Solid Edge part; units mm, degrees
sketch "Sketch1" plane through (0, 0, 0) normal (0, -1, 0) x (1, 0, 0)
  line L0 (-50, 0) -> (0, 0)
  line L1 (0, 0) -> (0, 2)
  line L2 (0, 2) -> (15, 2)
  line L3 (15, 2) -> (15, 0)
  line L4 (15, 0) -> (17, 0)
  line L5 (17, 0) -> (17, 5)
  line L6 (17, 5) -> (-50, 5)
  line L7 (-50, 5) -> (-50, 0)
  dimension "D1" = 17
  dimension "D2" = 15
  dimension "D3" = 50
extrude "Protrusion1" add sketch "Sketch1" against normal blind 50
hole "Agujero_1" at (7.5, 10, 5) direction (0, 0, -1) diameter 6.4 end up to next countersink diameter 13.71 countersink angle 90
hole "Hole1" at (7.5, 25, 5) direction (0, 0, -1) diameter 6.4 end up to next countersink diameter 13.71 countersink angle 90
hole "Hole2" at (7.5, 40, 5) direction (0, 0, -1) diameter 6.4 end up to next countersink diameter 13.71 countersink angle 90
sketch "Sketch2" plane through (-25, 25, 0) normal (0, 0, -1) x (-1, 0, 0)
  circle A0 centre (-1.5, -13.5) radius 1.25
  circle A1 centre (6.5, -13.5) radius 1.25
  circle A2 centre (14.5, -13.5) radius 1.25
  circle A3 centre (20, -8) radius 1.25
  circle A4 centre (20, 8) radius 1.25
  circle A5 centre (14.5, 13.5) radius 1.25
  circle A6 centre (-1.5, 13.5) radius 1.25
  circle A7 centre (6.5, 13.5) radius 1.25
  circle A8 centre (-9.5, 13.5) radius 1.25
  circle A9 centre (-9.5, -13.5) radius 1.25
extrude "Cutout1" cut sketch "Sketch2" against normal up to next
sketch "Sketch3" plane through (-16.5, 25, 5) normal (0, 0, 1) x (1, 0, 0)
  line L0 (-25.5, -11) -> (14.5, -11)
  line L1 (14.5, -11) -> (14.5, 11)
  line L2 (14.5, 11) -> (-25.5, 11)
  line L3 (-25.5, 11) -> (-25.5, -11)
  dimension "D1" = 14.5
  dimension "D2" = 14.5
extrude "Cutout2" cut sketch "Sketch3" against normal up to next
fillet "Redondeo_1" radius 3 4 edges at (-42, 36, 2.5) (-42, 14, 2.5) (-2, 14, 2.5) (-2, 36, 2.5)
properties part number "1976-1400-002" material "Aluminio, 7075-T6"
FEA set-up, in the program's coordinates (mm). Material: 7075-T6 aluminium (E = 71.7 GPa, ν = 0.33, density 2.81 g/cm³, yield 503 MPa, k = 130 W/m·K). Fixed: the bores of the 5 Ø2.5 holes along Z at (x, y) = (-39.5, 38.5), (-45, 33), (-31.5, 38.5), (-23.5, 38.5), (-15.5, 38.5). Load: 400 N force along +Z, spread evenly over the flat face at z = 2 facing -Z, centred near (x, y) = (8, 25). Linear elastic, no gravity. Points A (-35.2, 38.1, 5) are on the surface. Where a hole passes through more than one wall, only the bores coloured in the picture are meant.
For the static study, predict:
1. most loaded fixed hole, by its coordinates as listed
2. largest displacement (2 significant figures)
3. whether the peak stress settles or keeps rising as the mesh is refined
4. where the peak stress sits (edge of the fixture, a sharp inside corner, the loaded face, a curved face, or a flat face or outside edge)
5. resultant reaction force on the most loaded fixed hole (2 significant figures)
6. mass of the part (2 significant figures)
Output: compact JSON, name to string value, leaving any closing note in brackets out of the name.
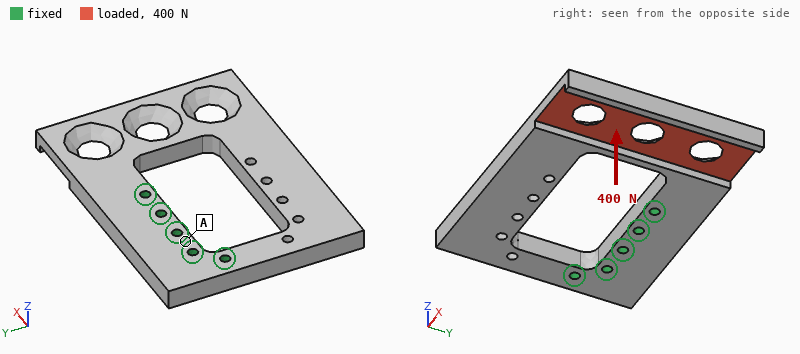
{"most loaded fixed hole, by its coordinates as listed": "(-15.5, 38.5)", "largest displacement": "0.89 mm", "whether the peak stress settles or keeps rising as the mesh is refined": "keeps rising", "where the peak stress sits": "edge of the fixture", "resultant reaction force on the most loaded fixed hole": "680 N", "mass of the part": "28 g"}
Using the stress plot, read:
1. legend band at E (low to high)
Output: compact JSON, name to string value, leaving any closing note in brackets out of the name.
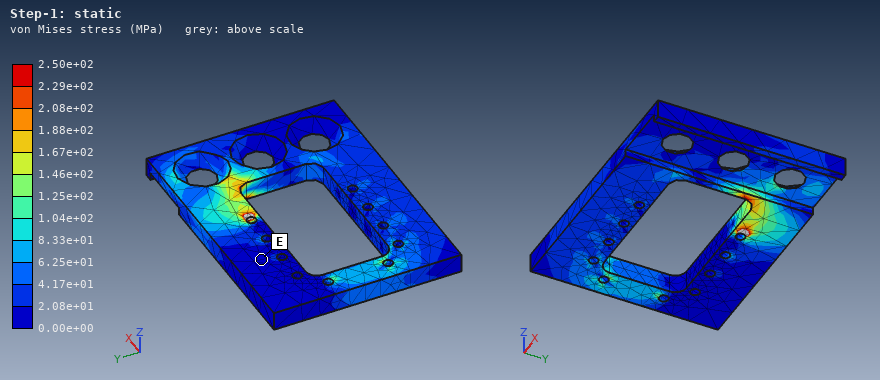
{"legend band at E": "0.00e+00 to 2.08e+01 MPa"}
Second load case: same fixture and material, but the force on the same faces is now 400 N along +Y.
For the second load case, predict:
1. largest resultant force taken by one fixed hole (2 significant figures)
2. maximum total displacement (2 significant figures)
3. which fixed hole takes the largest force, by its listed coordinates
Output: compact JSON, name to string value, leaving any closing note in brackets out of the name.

{"largest resultant force taken by one fixed hole": "820 N", "maximum total displacement": "55 µm", "which fixed hole takes the largest force, by its listed coordinates": "(-15.5, 38.5)"}
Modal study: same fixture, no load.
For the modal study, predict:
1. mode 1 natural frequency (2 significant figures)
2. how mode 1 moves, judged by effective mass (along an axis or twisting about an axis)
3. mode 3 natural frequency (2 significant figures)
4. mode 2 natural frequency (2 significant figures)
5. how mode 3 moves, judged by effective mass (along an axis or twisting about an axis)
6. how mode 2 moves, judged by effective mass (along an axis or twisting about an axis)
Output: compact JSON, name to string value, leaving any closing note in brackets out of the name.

{"mode 1 natural frequency": "1200 Hz", "how mode 1 moves, judged by effective mass": "along Z", "mode 3 natural frequency": "4000 Hz", "mode 2 natural frequency": "2600 Hz", "how mode 3 moves, judged by effective mass": "along X", "how mode 2 moves, judged by effective mass": "twisting about Y"}
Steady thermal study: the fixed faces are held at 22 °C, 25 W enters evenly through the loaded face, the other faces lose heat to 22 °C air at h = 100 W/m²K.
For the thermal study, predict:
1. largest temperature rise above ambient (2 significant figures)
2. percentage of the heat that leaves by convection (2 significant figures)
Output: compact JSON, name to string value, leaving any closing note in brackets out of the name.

{"largest temperature rise above ambient": "48 K", "percentage of the heat that leaves by convection": "47 %"}
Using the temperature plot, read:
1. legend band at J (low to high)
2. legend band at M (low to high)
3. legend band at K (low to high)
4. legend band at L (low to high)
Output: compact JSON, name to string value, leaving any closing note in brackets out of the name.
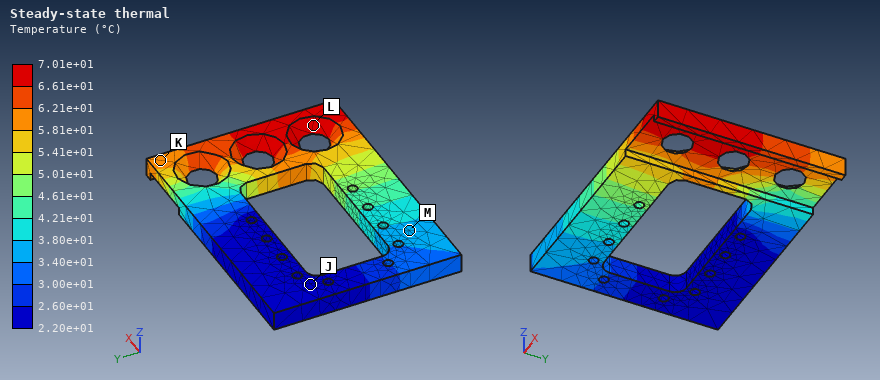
{"legend band at J": "2.20e+01 to 2.60e+01 °C", "legend band at M": "3.40e+01 to 3.80e+01 °C", "legend band at K": "5.81e+01 to 6.21e+01 °C", "legend band at L": "6.61e+01 to 7.01e+01 °C"}
